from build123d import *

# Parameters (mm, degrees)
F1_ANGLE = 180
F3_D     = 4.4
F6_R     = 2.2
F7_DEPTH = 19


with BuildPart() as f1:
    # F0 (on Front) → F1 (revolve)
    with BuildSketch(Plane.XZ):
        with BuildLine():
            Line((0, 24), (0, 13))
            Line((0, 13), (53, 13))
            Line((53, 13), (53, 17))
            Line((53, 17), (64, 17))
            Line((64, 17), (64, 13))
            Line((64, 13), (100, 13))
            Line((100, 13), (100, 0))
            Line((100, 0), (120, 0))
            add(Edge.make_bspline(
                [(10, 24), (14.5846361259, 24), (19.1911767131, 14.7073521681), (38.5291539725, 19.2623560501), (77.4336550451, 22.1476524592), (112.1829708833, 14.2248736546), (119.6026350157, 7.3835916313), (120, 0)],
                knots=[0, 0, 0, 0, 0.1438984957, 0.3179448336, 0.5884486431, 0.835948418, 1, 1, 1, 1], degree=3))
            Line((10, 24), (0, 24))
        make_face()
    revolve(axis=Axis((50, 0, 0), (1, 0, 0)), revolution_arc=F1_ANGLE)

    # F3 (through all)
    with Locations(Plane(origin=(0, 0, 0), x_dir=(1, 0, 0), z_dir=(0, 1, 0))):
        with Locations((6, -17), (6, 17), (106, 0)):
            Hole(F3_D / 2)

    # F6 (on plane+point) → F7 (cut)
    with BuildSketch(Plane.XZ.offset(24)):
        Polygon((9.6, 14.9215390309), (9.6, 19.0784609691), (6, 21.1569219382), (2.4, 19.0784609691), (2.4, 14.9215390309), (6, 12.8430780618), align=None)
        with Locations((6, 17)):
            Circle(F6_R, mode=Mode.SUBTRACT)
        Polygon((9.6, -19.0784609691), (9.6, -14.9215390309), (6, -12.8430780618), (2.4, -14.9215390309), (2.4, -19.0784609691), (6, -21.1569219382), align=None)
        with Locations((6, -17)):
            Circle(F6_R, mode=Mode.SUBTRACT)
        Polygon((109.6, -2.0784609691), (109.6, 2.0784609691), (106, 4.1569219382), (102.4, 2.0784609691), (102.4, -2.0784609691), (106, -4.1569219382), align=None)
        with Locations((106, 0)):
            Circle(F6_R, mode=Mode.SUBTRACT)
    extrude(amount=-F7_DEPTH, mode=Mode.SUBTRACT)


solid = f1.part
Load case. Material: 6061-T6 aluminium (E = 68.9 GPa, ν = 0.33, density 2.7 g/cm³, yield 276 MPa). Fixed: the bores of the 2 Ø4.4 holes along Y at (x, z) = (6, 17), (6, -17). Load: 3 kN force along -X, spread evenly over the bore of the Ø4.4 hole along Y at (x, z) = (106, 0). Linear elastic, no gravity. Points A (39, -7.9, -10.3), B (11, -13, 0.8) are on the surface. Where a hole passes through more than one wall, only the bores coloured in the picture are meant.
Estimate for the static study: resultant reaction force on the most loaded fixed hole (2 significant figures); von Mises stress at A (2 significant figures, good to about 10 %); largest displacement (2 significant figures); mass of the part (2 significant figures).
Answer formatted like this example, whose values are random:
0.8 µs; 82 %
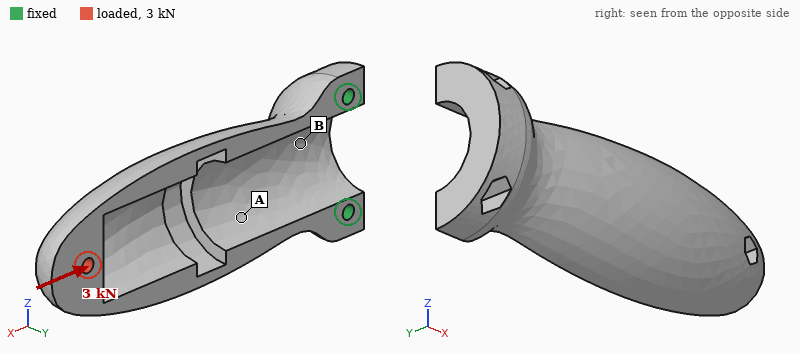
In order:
1.5 kN; 20 MPa; 0.38 mm; 99 g
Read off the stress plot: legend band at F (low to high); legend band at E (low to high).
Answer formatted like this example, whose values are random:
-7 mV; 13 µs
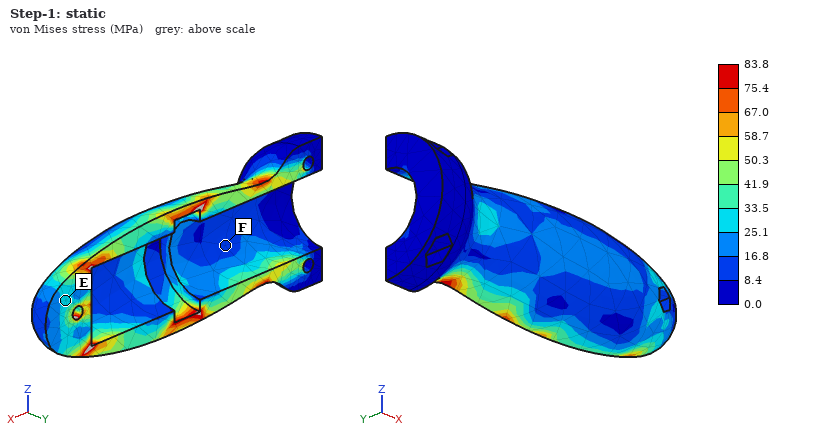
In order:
8.4 to 16.8 MPa; 25.1 to 33.5 MPa
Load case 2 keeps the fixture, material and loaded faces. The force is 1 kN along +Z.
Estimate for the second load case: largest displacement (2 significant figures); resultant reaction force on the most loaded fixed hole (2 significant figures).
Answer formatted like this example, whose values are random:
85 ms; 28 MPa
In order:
0.66 mm; 2.6 kN
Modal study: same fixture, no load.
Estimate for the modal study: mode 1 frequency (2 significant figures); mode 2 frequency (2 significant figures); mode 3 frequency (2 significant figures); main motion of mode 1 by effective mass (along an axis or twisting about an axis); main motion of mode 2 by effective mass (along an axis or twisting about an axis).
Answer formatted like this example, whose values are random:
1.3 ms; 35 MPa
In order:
680 Hz; 1300 Hz; 3400 Hz; along Y; along Z
